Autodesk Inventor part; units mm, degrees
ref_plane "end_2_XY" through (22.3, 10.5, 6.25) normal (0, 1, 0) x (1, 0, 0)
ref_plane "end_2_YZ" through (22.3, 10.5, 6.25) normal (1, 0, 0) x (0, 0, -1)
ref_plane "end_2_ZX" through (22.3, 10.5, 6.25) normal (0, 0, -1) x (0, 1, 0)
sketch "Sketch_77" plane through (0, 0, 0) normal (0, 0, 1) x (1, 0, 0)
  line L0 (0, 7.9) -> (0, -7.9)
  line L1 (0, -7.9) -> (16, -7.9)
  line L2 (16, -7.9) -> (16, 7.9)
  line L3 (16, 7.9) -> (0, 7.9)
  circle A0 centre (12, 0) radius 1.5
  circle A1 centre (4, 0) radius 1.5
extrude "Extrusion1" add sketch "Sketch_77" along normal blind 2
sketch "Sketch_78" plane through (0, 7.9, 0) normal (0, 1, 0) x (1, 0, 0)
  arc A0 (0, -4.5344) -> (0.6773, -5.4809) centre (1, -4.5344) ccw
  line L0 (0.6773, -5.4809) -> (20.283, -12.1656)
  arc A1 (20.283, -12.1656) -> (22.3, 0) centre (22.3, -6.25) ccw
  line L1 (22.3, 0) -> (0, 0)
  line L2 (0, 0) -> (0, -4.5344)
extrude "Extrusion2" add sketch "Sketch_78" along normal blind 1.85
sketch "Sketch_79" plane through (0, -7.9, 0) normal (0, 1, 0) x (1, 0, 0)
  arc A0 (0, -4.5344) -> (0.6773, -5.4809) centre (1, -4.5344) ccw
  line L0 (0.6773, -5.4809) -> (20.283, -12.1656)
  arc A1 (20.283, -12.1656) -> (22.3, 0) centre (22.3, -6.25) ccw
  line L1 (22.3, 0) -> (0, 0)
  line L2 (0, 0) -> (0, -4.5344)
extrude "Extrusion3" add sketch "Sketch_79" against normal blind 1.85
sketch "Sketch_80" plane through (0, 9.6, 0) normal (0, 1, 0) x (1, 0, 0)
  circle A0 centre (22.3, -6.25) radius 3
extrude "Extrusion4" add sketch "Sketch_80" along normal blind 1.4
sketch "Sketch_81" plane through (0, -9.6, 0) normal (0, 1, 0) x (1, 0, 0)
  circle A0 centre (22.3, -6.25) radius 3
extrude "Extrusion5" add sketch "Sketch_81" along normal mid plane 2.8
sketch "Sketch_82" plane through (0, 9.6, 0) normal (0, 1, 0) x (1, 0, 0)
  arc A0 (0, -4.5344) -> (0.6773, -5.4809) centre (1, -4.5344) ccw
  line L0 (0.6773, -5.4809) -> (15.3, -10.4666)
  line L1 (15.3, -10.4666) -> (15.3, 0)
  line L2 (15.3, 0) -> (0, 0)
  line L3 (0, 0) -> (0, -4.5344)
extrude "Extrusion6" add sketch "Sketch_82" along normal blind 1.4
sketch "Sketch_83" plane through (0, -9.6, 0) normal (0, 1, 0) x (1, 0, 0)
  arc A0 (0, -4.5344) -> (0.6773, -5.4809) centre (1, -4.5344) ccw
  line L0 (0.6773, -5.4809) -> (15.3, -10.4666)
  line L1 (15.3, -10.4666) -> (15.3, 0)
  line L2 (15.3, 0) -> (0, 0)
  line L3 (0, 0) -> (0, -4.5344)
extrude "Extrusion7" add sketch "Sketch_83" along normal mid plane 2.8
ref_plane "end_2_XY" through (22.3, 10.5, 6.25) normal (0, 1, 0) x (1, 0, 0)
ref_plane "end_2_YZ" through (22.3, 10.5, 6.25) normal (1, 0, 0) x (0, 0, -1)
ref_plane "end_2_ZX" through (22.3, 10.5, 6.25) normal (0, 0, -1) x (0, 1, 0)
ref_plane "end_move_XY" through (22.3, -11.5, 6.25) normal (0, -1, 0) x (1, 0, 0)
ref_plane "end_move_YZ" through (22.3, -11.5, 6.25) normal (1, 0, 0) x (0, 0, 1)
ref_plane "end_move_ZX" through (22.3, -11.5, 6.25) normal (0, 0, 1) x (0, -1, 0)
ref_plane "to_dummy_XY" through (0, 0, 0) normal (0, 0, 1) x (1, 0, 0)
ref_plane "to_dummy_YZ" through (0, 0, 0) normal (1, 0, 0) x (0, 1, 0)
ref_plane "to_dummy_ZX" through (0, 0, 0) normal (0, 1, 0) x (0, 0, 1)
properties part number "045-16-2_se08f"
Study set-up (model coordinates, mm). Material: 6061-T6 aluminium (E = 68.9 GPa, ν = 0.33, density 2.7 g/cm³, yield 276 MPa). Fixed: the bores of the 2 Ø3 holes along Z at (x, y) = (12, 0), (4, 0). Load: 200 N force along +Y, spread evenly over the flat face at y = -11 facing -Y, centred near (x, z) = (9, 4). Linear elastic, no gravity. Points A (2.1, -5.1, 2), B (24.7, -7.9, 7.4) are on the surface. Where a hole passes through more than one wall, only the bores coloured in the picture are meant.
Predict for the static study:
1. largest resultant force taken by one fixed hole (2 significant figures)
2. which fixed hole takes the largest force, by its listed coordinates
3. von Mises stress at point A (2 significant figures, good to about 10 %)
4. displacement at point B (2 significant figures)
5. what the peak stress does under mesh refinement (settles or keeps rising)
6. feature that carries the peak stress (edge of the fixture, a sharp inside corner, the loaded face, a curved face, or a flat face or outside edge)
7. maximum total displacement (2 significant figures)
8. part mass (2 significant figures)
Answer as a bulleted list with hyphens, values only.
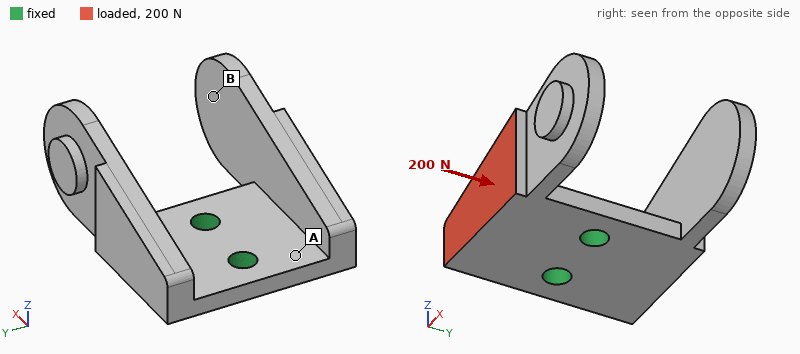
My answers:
- 110 N
- (12, 0)
- 56 MPa
- 47 µm
- keeps rising
- edge of the fixture
- 84 µm
- 4.9 g
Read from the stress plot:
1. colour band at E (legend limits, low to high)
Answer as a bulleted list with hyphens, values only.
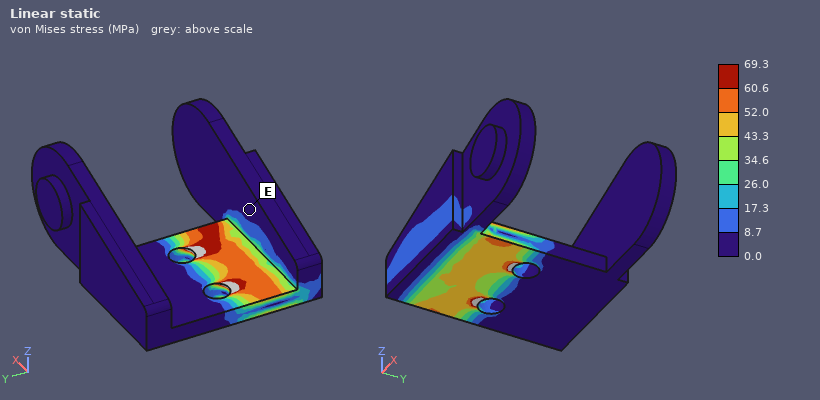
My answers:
- 0.0 to 8.7 MPa
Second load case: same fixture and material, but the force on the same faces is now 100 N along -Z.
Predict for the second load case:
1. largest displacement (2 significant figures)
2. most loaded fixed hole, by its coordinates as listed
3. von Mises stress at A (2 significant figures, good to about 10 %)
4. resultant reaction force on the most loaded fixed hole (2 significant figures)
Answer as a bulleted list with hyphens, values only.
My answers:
- 84 µm
- (12, 0)
- 50 MPa
- 55 N
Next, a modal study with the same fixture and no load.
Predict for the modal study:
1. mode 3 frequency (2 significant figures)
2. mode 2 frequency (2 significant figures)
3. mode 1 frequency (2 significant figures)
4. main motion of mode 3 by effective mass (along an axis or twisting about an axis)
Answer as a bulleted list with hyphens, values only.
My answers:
- 6600 Hz
- 4300 Hz
- 4300 Hz
- along Y
